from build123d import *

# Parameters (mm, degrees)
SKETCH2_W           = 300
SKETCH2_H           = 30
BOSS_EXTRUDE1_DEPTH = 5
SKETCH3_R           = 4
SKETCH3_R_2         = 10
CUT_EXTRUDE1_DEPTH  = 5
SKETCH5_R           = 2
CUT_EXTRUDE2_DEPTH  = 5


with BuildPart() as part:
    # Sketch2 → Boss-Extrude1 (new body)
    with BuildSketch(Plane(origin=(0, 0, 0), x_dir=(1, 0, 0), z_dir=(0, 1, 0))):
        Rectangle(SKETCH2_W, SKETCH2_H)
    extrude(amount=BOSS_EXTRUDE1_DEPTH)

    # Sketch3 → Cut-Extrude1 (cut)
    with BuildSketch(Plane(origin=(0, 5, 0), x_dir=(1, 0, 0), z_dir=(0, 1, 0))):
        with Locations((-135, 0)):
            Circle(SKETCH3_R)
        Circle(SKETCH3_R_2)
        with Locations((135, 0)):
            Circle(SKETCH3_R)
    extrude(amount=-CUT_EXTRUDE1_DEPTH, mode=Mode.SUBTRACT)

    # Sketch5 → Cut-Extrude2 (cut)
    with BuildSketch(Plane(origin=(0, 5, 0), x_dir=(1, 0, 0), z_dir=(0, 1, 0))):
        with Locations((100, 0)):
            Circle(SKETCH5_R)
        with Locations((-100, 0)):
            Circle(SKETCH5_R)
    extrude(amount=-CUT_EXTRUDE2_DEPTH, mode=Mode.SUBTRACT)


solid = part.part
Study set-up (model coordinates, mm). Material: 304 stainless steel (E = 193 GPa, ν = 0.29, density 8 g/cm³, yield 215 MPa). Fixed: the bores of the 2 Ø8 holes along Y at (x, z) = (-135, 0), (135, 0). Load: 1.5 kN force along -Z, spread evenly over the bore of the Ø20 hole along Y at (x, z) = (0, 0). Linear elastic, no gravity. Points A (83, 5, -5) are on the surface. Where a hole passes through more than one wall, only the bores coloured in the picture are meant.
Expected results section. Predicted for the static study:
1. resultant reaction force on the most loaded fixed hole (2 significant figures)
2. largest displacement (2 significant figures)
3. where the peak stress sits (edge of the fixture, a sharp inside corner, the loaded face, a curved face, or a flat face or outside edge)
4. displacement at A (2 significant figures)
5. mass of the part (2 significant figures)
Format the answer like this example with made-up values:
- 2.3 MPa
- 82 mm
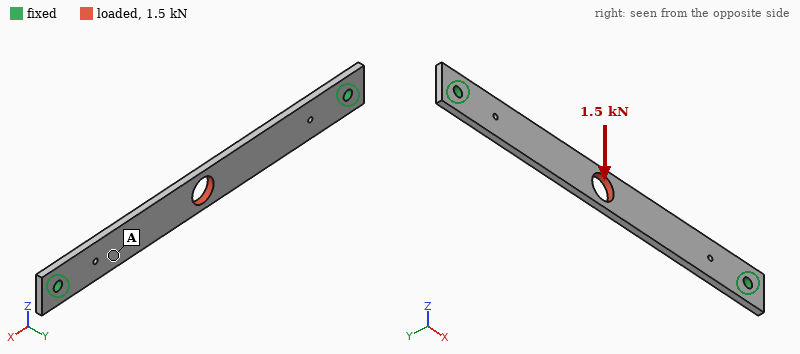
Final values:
- 750 N
- 0.12 mm
- edge of the fixture
- 0.048 mm
- 340 g
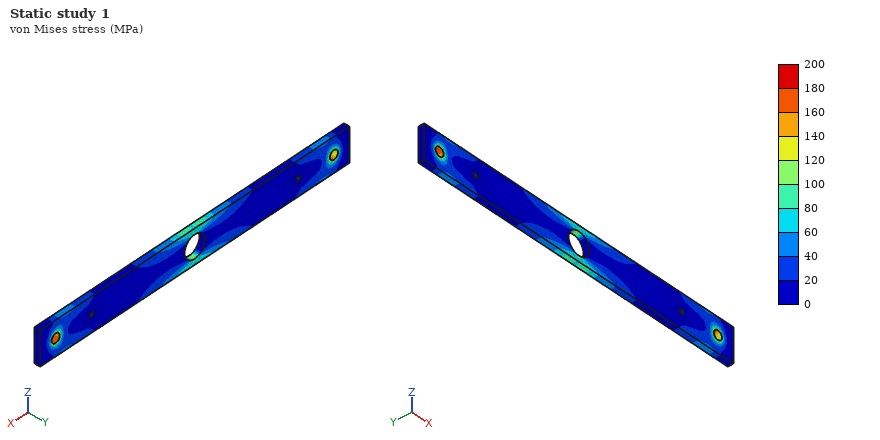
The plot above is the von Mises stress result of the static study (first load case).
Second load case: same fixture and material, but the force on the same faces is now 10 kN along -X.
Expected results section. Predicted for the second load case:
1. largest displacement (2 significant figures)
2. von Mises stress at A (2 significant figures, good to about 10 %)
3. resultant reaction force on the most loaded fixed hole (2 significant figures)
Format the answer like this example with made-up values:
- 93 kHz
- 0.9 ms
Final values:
- 24 µm
- 33 MPa
- 5.0 kN
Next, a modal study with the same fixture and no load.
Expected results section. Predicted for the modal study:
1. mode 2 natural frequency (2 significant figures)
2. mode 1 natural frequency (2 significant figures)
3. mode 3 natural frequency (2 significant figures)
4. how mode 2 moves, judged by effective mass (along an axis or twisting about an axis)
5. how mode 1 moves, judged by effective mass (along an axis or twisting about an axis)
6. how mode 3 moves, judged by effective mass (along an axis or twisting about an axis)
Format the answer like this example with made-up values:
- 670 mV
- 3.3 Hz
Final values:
- 970 Hz
- 350 Hz
- 1600 Hz
- twisting about Z
- along Y
- along Z
